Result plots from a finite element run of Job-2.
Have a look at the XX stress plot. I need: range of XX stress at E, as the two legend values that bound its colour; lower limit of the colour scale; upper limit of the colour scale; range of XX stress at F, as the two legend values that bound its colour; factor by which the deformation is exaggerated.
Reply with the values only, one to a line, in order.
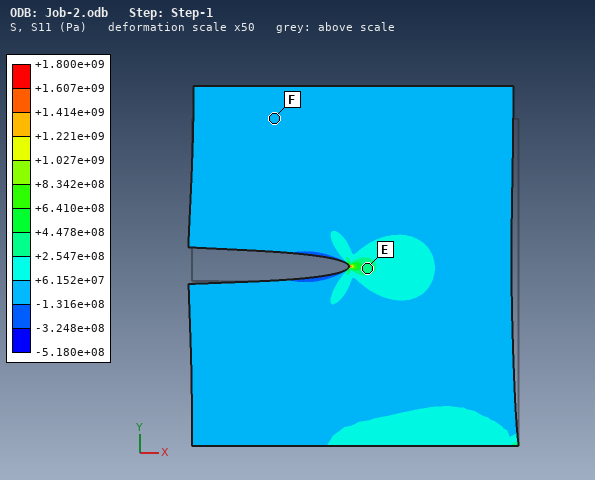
+2.547e+08 to +4.478e+08 Pa
-5.180e+08 Pa
+1.800e+09 Pa
-1.316e+08 to +6.152e+07 Pa
50
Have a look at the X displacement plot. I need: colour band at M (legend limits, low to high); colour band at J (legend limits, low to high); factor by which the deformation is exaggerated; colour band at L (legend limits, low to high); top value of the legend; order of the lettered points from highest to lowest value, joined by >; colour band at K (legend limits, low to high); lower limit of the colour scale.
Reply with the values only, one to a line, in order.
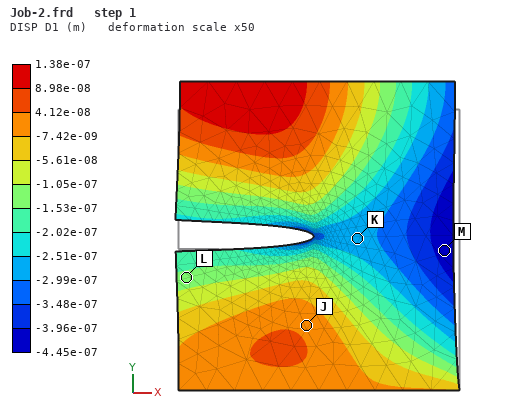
-4.45e-07 to -3.96e-07 m
-7.42e-09 to 4.12e-08 m
50
-1.53e-07 to -1.05e-07 m
1.38e-07 m
J > L > K > M
-2.99e-07 to -2.51e-07 m
-4.45e-07 m
